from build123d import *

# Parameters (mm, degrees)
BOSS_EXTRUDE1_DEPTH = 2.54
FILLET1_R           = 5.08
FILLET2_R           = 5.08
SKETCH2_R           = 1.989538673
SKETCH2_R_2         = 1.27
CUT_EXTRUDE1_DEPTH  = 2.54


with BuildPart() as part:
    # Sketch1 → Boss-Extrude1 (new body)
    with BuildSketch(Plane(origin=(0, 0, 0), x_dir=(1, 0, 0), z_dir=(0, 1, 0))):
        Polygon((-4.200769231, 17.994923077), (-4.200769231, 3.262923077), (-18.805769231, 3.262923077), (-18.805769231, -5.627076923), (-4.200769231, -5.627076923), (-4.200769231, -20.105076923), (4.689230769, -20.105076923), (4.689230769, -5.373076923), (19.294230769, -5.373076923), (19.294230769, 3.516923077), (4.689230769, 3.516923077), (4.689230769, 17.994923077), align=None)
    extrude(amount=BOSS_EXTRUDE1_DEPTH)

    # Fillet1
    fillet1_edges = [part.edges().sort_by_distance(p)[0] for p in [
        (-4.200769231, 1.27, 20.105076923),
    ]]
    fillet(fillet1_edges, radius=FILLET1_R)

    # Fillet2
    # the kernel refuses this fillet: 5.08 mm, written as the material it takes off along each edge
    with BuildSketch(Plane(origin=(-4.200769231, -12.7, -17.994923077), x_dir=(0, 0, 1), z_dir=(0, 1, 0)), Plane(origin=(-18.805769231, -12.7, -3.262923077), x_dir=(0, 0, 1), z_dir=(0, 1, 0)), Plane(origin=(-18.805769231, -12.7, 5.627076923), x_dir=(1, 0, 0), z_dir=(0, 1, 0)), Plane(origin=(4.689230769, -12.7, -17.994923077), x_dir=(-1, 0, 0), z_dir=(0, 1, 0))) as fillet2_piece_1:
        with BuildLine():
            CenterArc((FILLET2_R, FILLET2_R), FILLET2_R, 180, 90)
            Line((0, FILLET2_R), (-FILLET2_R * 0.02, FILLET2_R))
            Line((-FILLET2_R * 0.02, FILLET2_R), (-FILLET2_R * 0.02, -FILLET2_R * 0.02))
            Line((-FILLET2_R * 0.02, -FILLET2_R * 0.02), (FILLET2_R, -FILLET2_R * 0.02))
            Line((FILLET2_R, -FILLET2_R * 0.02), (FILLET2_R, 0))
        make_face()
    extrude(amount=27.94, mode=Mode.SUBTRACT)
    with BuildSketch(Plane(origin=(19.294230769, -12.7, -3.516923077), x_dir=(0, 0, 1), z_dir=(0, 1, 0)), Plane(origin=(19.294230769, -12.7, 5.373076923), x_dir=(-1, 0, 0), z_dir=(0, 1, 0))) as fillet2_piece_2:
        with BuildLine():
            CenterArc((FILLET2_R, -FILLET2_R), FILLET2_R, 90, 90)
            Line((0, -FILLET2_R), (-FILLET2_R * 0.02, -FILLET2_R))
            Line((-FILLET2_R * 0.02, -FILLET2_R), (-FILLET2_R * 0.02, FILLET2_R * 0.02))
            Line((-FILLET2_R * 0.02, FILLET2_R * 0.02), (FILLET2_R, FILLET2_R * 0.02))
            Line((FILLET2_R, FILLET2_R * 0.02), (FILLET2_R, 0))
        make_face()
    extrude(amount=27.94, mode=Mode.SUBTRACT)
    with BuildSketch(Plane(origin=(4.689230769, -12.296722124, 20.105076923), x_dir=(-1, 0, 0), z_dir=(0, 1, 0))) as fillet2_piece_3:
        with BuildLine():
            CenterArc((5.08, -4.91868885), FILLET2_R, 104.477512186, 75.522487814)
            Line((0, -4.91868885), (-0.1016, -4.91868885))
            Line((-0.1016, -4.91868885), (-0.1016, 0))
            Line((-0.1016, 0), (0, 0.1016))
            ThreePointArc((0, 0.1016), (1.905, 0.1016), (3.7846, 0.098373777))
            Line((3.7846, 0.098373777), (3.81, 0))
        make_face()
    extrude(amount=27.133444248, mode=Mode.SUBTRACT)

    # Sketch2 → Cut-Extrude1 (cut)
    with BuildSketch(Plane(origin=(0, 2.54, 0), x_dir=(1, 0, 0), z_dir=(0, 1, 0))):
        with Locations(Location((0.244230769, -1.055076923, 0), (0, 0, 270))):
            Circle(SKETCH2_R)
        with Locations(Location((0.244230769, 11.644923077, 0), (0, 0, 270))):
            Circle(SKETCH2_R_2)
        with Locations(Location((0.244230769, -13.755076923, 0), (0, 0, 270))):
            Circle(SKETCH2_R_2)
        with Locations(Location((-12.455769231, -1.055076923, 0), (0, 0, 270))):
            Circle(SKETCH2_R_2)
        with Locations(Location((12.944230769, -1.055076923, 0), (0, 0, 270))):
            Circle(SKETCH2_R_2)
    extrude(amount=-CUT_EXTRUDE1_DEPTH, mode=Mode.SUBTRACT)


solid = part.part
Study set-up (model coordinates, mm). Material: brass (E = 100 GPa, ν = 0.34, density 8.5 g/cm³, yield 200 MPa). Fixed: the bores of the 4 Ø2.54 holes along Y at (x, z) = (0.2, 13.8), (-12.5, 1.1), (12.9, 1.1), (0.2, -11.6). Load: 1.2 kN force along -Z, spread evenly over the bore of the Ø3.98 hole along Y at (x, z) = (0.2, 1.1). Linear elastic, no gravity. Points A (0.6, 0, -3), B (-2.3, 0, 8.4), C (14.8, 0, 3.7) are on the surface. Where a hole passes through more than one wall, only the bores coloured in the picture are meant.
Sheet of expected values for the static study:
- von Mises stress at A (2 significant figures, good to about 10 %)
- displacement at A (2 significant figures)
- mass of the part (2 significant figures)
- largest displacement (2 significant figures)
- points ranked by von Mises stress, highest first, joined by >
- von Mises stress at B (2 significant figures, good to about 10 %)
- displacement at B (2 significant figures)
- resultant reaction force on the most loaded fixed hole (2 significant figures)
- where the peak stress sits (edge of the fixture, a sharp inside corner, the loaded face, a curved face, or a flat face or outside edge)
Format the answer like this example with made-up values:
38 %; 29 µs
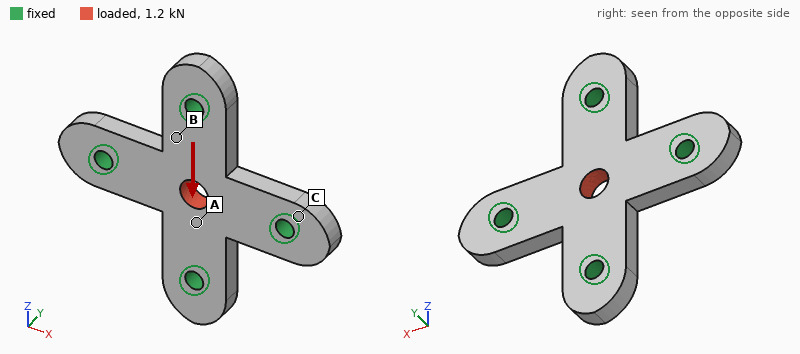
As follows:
39 MPa; 2.5 µm; 11 g; 3.6 µm; A > B > C; 23 MPa; 1.5 µm; 530 N; the loaded face
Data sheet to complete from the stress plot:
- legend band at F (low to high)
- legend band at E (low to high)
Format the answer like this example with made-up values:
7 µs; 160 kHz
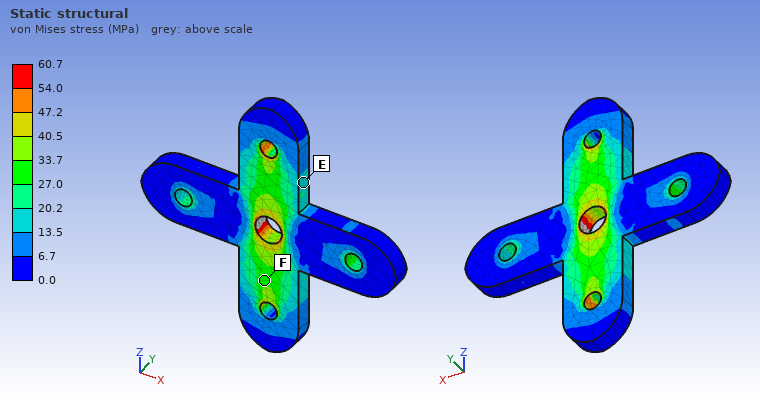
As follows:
27.0 to 33.7 MPa; 13.5 to 20.2 MPa
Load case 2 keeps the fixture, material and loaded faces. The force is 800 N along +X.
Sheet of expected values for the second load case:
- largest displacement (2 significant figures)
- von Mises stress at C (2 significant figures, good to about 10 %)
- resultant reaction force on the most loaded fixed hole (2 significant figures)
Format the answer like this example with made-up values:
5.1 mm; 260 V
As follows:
2.4 µm; 6.1 MPa; 360 N
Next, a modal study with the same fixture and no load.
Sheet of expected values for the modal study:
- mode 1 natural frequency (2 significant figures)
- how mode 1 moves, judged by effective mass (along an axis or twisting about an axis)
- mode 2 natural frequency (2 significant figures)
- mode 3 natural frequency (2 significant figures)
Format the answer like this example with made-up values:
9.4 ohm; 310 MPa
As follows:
19 kHz; along Y; 35 kHz; 35 kHz
